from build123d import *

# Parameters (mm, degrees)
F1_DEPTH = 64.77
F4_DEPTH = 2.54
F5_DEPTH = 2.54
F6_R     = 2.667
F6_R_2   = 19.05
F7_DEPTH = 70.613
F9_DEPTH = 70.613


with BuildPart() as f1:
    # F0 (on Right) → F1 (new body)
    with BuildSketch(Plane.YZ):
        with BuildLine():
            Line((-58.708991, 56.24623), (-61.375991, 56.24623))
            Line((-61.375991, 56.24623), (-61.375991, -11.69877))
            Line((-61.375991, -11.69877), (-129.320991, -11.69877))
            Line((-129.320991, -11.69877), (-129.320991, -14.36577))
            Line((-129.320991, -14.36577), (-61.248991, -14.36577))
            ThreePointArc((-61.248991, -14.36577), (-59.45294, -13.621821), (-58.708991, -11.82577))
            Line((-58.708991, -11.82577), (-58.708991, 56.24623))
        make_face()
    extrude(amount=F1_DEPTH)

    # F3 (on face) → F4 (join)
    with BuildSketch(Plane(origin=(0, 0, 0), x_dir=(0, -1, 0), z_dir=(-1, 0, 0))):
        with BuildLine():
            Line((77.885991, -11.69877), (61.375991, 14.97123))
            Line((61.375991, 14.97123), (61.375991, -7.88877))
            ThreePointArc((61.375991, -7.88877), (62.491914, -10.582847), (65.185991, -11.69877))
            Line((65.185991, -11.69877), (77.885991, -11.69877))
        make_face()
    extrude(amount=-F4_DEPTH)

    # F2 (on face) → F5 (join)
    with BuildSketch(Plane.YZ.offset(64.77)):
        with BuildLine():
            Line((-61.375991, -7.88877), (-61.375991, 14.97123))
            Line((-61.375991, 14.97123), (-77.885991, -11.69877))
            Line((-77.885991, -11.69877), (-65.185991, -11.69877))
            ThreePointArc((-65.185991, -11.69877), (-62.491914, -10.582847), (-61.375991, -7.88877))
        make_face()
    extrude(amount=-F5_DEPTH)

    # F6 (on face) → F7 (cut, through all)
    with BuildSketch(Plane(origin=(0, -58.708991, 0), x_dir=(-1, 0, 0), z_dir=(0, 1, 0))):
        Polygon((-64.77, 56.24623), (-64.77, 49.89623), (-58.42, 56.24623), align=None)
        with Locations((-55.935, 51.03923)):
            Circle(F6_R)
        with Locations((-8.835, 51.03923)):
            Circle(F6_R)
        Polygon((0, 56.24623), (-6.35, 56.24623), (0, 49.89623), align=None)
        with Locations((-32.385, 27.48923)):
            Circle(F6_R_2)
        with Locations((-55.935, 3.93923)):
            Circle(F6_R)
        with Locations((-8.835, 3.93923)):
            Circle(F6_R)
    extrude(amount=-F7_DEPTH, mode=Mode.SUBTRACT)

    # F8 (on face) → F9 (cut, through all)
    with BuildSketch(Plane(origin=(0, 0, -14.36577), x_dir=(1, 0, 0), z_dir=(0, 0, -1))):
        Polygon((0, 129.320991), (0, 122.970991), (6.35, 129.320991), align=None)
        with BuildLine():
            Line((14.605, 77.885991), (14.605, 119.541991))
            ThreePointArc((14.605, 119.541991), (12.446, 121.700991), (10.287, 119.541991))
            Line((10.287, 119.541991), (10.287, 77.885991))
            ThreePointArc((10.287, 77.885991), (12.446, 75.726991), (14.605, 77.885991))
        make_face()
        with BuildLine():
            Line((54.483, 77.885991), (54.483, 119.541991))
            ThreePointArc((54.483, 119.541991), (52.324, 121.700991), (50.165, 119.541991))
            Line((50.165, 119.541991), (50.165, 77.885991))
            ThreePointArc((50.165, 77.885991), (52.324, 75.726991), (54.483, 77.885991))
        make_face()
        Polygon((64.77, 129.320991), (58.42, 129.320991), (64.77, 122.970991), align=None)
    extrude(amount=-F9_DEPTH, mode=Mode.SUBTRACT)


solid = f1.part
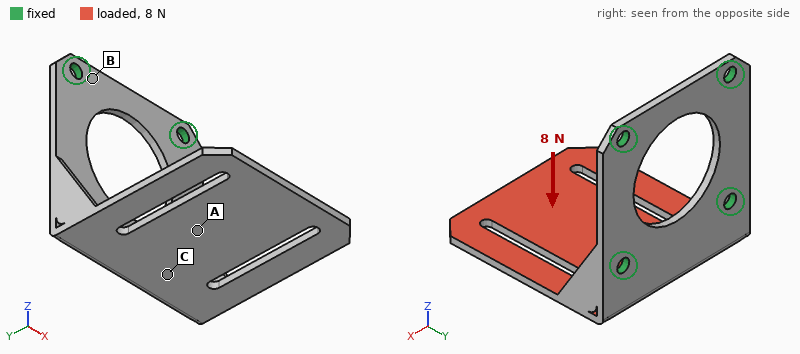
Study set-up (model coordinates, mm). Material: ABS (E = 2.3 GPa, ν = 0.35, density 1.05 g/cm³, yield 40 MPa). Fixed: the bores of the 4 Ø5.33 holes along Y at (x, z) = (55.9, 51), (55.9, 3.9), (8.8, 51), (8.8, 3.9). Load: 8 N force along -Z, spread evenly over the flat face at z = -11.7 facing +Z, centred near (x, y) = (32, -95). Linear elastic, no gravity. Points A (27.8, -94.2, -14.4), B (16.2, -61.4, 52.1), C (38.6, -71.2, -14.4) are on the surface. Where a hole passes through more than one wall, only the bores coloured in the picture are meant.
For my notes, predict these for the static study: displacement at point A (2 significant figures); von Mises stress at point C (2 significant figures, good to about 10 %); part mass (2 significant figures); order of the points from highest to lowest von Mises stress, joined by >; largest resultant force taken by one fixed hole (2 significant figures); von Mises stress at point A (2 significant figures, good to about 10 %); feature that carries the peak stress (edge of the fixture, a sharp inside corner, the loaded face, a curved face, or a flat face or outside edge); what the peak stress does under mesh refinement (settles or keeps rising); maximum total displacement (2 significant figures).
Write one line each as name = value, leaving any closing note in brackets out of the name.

displacement at point A = 0.51 mm
von Mises stress at point C = 1.4 MPa
part mass = 21 g
order of the points from highest to lowest von Mises stress, joined by > = C > A > B
largest resultant force taken by one fixed hole = 4.6 N
von Mises stress at point A = 0.88 MPa
feature that carries the peak stress = edge of the fixture
what the peak stress does under mesh refinement = keeps rising
maximum total displacement = 1.4 mm
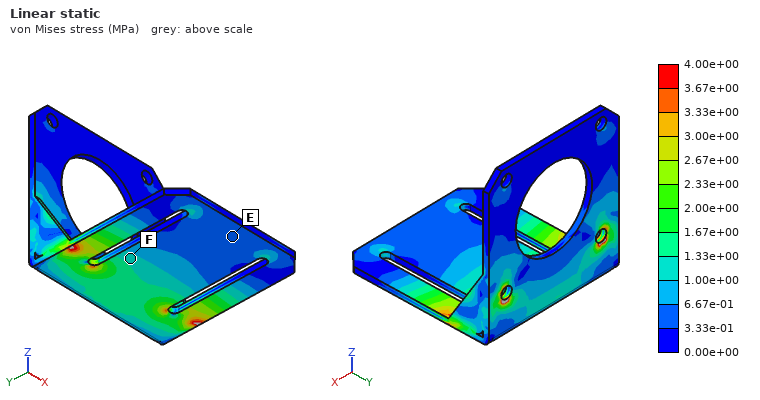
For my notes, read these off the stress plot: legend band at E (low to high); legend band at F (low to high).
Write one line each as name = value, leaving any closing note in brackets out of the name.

legend band at E = 3.33e-01 to 6.67e-01 MPa
legend band at F = 1.00e+00 to 1.33e+00 MPa
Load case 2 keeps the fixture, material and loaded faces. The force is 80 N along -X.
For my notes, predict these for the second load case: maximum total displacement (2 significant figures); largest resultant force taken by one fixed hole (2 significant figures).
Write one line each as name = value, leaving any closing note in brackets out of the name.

maximum total displacement = 1.3 mm
largest resultant force taken by one fixed hole = 74 N
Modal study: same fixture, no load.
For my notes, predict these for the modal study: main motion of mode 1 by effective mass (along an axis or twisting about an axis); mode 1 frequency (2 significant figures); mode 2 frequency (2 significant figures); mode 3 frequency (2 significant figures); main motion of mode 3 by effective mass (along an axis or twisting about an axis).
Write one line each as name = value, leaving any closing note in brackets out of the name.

main motion of mode 1 by effective mass = along Z
mode 1 frequency = 150 Hz
mode 2 frequency = 370 Hz
mode 3 frequency = 560 Hz
main motion of mode 3 by effective mass = along X
